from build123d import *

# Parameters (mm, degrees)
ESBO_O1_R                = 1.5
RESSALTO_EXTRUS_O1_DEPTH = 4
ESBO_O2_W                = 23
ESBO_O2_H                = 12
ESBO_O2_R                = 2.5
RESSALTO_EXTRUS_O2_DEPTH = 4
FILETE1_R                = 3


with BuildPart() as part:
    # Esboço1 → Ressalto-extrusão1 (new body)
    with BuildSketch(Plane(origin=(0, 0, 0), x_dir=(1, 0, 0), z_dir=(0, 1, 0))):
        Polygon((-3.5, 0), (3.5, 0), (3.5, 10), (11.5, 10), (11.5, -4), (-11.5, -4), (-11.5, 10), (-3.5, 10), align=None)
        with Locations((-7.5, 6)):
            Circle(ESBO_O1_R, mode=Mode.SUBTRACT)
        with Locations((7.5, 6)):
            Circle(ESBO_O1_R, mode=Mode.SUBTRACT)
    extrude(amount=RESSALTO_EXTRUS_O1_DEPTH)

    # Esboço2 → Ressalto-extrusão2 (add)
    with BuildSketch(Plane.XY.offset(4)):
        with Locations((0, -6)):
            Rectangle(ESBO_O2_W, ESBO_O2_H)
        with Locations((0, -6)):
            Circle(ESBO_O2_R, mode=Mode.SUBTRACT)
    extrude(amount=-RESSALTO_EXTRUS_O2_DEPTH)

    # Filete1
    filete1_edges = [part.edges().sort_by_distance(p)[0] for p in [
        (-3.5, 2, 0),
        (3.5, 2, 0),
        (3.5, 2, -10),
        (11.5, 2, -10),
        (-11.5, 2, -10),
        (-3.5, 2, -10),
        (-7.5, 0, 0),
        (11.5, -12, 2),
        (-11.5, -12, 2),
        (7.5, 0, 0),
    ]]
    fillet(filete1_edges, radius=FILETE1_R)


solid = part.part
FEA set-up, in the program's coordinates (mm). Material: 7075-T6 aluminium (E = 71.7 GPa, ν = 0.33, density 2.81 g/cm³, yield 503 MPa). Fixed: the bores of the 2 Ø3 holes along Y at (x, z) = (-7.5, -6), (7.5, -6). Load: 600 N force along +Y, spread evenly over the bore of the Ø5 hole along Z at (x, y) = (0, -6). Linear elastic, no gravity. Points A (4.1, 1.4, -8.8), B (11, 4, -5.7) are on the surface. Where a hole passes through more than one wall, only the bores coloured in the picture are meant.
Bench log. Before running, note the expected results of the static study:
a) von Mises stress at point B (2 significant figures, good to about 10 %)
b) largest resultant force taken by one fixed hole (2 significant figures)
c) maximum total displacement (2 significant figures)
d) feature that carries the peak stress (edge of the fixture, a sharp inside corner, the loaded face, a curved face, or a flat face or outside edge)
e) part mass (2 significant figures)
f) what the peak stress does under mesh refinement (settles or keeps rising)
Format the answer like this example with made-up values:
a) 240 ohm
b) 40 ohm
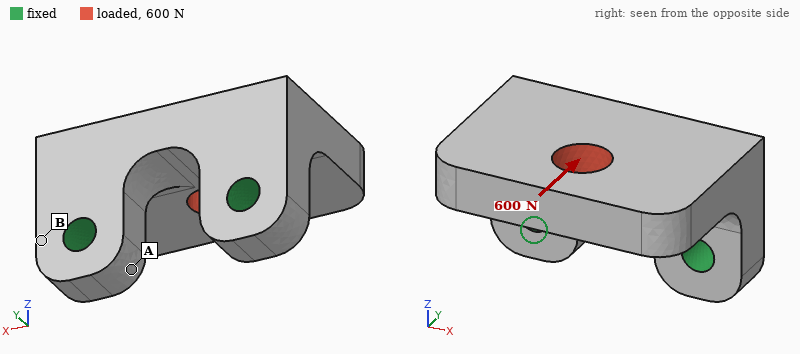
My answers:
a) 38 MPa
b) 300 N
c) 42 µm
d) edge of the fixture
e) 5.6 g
f) keeps rising
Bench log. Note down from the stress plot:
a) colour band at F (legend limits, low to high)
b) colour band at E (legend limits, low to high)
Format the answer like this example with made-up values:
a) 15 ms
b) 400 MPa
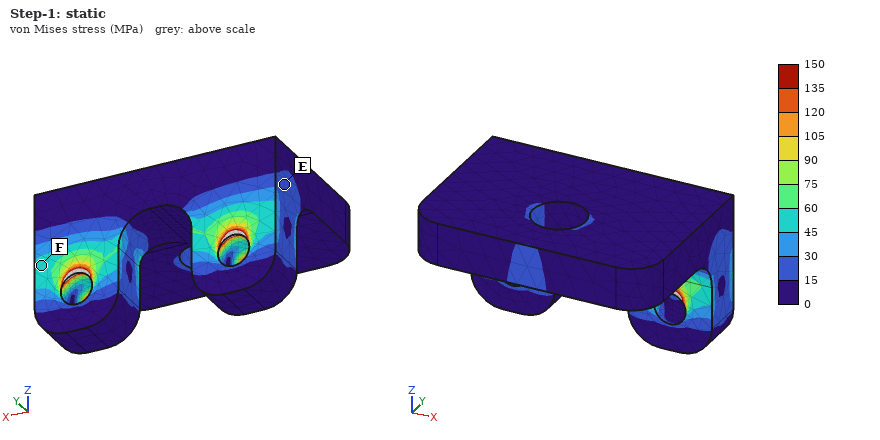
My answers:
a) 45 to 60 MPa
b) 15 to 30 MPa
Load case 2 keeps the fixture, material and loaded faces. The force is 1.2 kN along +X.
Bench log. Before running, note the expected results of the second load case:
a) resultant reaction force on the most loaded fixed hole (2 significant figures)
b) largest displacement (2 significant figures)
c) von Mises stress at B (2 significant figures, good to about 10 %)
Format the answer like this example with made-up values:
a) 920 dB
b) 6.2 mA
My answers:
a) 880 N
b) 39 µm
c) 62 MPa
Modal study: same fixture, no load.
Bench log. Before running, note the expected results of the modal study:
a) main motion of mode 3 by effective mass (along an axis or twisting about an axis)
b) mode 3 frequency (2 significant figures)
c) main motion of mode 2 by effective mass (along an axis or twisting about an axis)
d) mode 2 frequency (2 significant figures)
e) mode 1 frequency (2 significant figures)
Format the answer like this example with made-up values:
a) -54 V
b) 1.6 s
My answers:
a) along X
b) 25 kHz
c) along X
d) 16 kHz
e) 9000 Hz
